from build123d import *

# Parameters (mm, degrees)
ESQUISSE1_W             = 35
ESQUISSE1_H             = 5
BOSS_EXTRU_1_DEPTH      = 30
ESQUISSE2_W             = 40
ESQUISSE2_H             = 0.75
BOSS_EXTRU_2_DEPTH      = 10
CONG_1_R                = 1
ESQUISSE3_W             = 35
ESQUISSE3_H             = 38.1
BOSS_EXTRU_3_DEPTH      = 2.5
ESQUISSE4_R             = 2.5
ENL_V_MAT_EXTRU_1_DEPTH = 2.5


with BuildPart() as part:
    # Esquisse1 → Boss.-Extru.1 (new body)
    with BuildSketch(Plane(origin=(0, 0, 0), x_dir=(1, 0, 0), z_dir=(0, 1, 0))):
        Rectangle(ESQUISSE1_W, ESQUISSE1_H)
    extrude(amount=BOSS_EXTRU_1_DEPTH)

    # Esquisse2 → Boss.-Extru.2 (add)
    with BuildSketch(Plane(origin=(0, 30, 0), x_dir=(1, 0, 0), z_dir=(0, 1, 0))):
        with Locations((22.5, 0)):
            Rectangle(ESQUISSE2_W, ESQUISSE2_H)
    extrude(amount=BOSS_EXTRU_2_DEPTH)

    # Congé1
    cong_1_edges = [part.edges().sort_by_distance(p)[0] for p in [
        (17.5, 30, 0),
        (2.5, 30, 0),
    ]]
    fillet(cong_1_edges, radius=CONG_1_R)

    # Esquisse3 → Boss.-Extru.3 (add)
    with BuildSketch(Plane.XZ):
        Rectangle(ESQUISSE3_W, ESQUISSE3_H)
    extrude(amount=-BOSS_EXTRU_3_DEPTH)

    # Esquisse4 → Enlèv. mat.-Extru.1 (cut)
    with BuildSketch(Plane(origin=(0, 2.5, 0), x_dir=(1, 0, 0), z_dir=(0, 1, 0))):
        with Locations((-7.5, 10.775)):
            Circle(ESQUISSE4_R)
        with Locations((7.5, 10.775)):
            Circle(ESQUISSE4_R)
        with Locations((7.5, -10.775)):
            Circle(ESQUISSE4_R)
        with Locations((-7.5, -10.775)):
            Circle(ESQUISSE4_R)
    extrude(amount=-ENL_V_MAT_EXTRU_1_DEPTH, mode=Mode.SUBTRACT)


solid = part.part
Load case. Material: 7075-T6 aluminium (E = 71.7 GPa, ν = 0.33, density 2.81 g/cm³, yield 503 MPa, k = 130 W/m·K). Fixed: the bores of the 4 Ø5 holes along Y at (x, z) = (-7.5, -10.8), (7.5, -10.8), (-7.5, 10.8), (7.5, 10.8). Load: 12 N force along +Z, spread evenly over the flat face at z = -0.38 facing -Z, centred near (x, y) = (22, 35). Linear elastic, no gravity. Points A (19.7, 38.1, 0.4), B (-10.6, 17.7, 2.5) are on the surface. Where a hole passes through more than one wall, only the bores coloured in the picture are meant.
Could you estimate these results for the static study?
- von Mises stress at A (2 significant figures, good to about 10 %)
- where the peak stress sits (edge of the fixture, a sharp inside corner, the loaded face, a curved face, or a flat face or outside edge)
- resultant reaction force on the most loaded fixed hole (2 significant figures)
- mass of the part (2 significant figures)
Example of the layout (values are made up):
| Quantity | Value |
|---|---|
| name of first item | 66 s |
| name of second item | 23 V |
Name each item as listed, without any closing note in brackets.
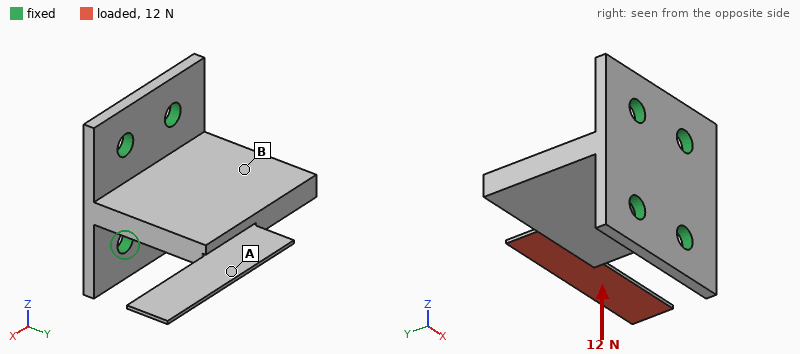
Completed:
| Quantity | Value |
|---|---|
| von Mises stress at A | 68 MPa |
| where the peak stress sits | a curved face |
| resultant reaction force on the most loaded fixed hole | 20 N |
| mass of the part | 23 g |
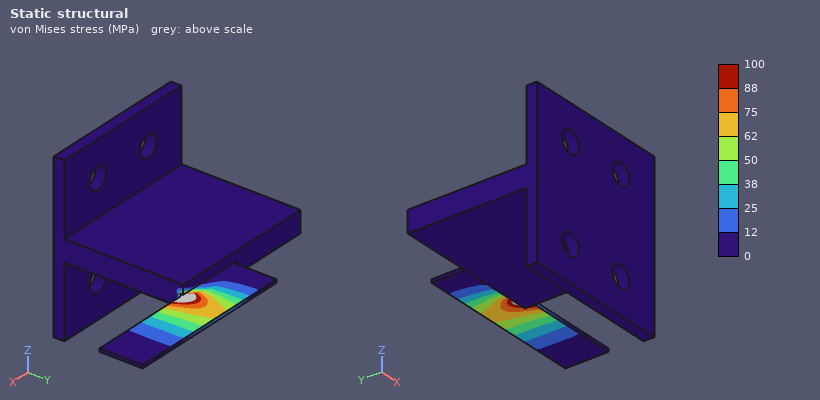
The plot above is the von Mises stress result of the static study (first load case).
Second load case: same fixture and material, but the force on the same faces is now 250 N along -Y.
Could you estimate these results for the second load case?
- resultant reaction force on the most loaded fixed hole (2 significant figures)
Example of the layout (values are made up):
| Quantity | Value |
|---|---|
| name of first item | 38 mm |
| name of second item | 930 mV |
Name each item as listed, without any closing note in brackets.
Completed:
| Quantity | Value |
|---|---|
| resultant reaction force on the most loaded fixed hole | 210 N |
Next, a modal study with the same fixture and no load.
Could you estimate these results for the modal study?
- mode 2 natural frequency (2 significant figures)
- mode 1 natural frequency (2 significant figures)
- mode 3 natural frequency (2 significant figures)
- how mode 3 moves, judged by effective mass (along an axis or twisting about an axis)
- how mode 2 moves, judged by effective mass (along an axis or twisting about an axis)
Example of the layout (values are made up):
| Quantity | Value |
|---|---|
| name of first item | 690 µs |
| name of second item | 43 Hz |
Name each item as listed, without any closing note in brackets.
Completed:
| Quantity | Value |
|---|---|
| mode 2 natural frequency | 3100 Hz |
| mode 1 natural frequency | 780 Hz |
| mode 3 natural frequency | 3800 Hz |
| how mode 3 moves, judged by effective mass | along Z |
| how mode 2 moves, judged by effective mass | along Z |
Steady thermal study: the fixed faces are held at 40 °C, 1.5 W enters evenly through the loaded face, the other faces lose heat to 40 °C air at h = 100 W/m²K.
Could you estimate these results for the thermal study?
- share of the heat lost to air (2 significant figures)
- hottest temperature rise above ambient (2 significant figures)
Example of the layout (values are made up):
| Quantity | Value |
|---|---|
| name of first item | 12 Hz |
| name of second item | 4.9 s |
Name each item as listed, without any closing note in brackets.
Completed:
| Quantity | Value |
|---|---|
| share of the heat lost to air | 44 % |
| hottest temperature rise above ambient | 14 K |
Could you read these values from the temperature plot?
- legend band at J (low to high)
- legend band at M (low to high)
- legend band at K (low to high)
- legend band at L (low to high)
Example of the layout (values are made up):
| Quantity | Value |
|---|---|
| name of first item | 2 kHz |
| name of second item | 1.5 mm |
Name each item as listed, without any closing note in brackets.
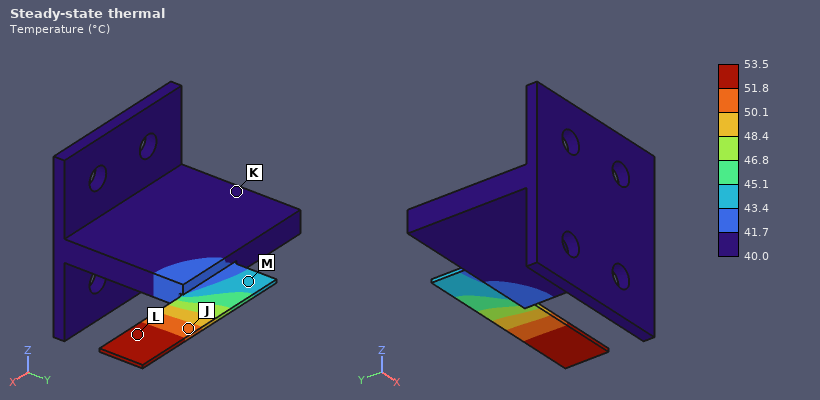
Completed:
| Quantity | Value |
|---|---|
| legend band at J | 50.1 to 51.8 °C |
| legend band at M | 43.4 to 45.1 °C |
| legend band at K | 40.0 to 41.7 °C |
| legend band at L | 51.8 to 53.5 °C |
